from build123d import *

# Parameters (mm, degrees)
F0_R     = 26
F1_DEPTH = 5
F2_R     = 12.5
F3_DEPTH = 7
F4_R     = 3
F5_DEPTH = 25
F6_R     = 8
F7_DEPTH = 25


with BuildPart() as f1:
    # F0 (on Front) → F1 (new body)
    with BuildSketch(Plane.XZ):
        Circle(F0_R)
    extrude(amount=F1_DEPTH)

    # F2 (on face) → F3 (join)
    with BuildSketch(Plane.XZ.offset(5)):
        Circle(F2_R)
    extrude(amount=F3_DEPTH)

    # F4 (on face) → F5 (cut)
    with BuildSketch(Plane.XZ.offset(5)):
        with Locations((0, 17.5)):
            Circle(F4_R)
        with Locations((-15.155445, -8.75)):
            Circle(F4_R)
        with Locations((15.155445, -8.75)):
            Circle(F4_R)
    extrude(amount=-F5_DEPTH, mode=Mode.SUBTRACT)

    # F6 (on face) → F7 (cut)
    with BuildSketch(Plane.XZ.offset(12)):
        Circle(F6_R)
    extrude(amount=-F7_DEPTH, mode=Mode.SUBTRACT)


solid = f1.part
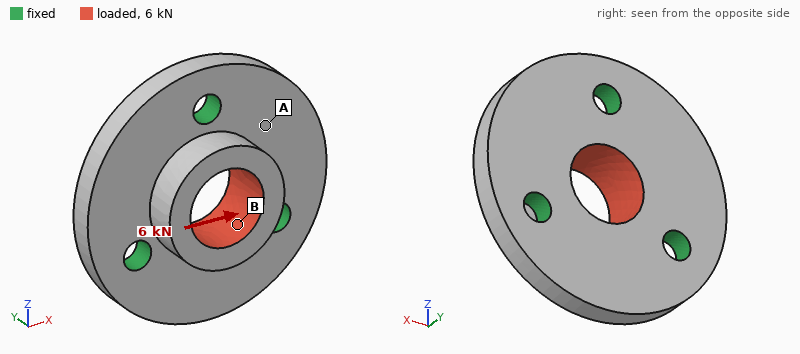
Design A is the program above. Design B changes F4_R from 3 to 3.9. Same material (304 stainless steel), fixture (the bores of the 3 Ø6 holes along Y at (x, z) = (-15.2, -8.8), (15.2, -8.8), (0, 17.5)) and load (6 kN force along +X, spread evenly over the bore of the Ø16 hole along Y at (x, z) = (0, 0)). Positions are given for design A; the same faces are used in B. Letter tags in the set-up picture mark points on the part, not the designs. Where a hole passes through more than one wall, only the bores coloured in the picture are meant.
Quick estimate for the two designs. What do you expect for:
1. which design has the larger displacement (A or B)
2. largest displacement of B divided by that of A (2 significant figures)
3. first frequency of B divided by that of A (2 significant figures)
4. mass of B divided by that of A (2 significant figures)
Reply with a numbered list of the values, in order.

1. A
2. 0.87
3. 1.1
4. 0.97
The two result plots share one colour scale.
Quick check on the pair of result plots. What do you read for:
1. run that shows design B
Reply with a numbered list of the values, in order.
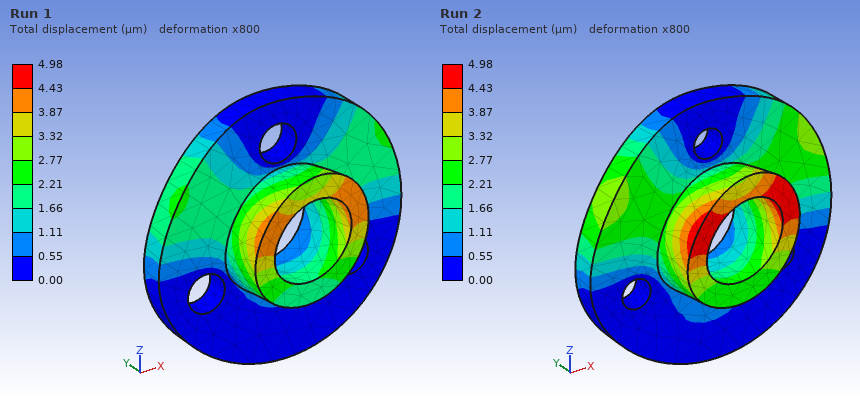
1. Run 1
